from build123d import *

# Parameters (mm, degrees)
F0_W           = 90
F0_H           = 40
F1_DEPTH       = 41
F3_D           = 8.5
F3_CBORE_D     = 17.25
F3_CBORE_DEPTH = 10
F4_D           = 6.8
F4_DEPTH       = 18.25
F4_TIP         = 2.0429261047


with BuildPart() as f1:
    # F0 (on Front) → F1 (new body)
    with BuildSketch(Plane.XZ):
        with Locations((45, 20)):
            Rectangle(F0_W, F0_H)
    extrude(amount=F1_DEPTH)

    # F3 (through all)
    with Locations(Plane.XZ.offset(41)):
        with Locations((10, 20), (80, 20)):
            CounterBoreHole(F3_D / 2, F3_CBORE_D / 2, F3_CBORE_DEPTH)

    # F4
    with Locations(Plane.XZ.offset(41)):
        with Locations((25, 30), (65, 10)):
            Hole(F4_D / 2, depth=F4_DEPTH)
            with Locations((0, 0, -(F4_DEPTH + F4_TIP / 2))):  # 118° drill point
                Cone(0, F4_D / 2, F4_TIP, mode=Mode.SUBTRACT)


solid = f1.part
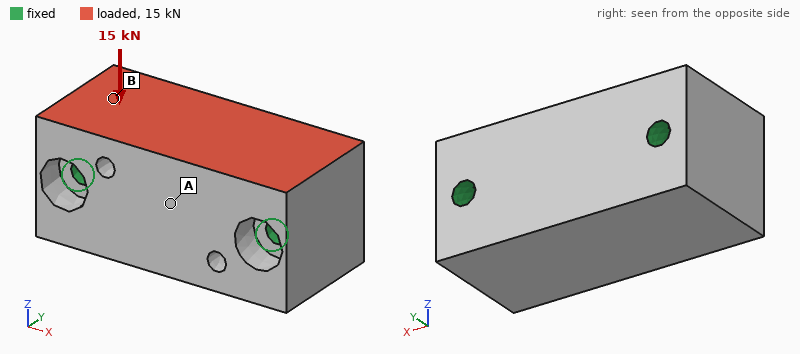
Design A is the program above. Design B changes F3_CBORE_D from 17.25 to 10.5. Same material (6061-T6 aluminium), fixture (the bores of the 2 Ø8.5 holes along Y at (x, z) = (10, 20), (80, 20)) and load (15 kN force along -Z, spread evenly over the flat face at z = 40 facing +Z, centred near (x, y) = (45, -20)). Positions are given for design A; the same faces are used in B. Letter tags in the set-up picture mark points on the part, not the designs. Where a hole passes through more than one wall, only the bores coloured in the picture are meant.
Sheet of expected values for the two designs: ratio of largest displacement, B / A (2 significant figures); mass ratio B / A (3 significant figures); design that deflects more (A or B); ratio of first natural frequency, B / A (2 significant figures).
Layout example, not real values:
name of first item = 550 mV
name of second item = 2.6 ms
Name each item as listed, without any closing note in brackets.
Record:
ratio of largest displacement, B / A = 0.91
mass ratio B / A = 1.02
design that deflects more = A
ratio of first natural frequency, B / A = 1.0
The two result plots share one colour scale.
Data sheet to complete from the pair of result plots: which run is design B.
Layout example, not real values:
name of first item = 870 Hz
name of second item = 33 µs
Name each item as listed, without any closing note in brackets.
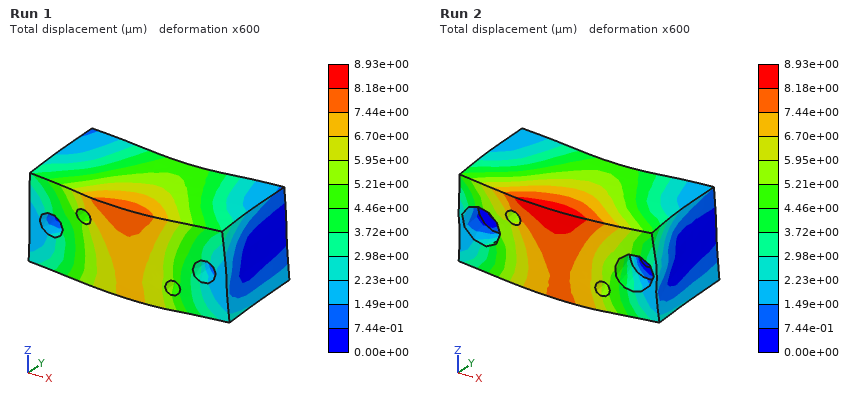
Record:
which run is design B = Run 1
